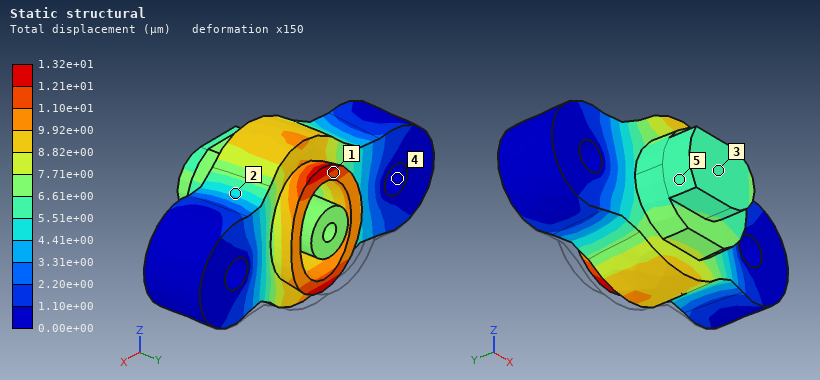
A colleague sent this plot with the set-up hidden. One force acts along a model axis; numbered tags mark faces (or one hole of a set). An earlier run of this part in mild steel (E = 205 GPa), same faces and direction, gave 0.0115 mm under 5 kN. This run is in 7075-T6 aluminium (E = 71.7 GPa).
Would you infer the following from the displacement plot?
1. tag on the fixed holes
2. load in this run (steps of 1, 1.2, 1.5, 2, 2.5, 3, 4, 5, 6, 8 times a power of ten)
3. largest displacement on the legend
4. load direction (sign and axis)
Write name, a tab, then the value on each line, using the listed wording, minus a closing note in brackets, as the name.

tag on the fixed holes	4
load in this run	2 kN
largest displacement on the legend	1.32e+01 µm
load direction	-Y
